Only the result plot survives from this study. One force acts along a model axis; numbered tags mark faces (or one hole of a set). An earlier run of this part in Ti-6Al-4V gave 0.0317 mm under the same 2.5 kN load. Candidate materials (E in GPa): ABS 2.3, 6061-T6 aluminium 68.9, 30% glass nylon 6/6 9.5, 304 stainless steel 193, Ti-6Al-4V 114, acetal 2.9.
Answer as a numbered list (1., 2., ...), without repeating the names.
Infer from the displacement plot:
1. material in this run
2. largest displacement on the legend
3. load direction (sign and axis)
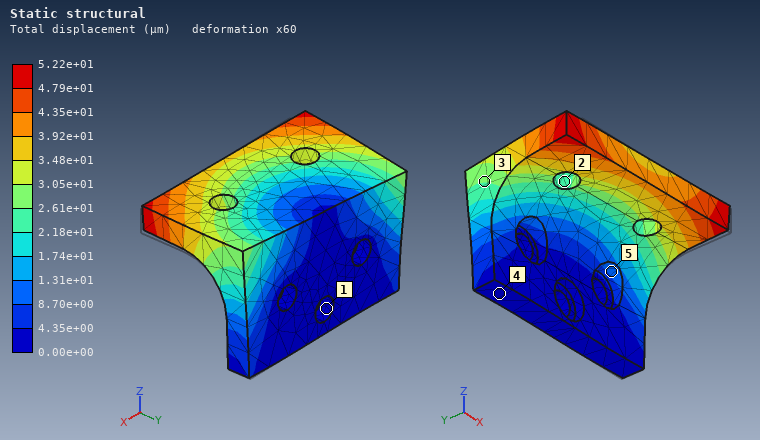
1. 6061-T6 aluminium
2. 5.22e+01 µm
3. -X
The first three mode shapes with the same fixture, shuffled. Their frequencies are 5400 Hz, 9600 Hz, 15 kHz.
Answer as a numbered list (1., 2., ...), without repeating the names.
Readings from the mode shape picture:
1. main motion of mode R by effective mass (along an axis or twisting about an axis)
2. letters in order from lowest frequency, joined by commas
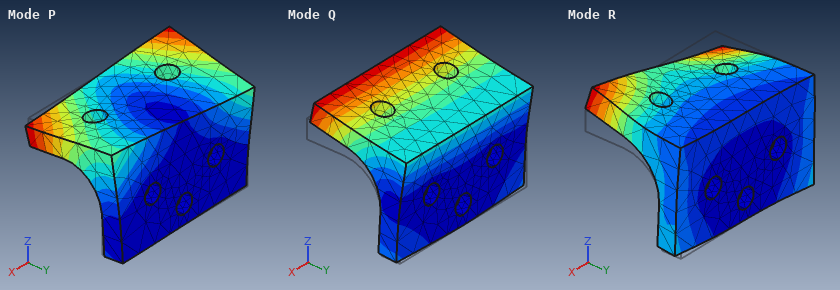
1. along X
2. Q, P, R
